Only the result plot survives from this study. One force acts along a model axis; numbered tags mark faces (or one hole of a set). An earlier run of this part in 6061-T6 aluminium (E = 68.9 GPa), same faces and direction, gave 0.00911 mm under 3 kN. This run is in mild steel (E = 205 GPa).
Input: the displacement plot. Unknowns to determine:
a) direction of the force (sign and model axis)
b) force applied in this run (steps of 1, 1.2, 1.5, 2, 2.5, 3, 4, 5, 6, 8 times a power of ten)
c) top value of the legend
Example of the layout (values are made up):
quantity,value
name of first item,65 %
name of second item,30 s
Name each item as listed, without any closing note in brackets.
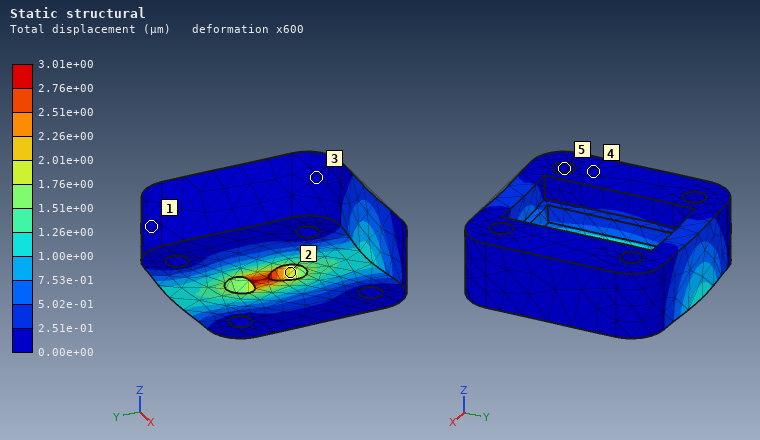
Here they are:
quantity,value
direction of the force,+Y
force applied in this run,3 kN
top value of the legend,3.01e+00 µm
